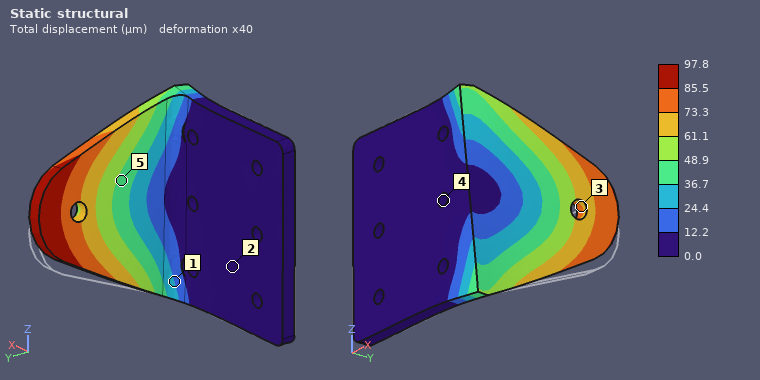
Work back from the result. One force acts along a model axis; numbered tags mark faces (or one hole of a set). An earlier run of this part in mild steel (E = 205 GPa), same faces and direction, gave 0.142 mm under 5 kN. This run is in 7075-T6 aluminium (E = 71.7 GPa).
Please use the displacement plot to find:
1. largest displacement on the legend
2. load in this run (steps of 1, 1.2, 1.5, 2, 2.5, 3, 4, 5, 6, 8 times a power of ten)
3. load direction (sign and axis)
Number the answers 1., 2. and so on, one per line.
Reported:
1. 97.8 µm
2. 1.2 kN
3. +Z
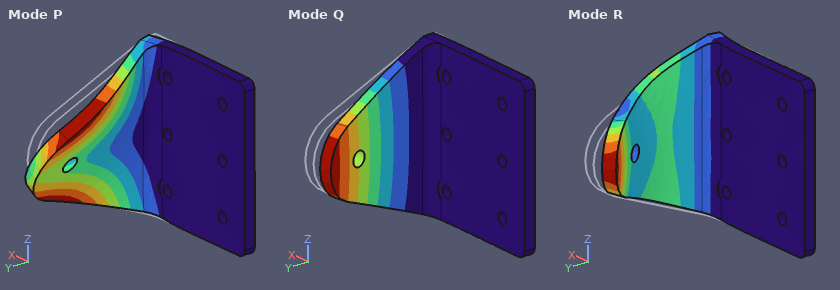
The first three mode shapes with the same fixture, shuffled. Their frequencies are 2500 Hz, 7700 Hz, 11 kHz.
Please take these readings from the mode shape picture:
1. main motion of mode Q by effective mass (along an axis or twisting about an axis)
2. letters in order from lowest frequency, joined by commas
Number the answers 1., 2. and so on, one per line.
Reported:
1. along X
2. Q, P, R
